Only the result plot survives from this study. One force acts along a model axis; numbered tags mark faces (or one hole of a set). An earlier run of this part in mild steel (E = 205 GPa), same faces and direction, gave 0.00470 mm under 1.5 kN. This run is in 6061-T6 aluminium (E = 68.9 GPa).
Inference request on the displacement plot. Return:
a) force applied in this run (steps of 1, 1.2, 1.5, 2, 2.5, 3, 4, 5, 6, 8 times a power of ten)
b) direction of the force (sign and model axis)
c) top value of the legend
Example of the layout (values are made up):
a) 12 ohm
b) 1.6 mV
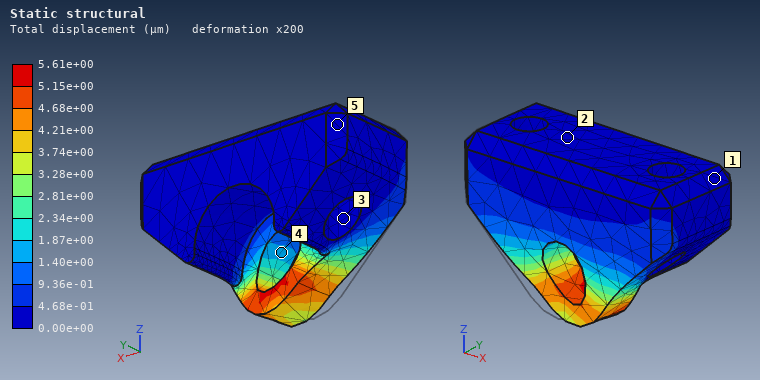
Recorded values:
a) 600 N
b) +X
c) 5.61e+00 µm
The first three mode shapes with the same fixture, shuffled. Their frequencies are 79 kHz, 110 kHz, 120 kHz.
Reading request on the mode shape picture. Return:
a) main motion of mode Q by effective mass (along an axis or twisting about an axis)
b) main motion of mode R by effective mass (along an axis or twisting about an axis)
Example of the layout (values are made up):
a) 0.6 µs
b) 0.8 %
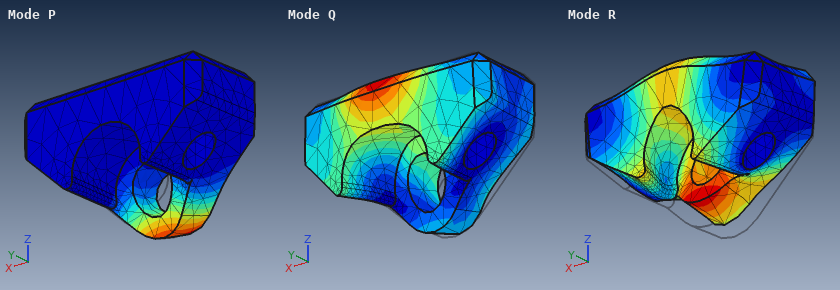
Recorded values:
a) along Y
b) along Z
